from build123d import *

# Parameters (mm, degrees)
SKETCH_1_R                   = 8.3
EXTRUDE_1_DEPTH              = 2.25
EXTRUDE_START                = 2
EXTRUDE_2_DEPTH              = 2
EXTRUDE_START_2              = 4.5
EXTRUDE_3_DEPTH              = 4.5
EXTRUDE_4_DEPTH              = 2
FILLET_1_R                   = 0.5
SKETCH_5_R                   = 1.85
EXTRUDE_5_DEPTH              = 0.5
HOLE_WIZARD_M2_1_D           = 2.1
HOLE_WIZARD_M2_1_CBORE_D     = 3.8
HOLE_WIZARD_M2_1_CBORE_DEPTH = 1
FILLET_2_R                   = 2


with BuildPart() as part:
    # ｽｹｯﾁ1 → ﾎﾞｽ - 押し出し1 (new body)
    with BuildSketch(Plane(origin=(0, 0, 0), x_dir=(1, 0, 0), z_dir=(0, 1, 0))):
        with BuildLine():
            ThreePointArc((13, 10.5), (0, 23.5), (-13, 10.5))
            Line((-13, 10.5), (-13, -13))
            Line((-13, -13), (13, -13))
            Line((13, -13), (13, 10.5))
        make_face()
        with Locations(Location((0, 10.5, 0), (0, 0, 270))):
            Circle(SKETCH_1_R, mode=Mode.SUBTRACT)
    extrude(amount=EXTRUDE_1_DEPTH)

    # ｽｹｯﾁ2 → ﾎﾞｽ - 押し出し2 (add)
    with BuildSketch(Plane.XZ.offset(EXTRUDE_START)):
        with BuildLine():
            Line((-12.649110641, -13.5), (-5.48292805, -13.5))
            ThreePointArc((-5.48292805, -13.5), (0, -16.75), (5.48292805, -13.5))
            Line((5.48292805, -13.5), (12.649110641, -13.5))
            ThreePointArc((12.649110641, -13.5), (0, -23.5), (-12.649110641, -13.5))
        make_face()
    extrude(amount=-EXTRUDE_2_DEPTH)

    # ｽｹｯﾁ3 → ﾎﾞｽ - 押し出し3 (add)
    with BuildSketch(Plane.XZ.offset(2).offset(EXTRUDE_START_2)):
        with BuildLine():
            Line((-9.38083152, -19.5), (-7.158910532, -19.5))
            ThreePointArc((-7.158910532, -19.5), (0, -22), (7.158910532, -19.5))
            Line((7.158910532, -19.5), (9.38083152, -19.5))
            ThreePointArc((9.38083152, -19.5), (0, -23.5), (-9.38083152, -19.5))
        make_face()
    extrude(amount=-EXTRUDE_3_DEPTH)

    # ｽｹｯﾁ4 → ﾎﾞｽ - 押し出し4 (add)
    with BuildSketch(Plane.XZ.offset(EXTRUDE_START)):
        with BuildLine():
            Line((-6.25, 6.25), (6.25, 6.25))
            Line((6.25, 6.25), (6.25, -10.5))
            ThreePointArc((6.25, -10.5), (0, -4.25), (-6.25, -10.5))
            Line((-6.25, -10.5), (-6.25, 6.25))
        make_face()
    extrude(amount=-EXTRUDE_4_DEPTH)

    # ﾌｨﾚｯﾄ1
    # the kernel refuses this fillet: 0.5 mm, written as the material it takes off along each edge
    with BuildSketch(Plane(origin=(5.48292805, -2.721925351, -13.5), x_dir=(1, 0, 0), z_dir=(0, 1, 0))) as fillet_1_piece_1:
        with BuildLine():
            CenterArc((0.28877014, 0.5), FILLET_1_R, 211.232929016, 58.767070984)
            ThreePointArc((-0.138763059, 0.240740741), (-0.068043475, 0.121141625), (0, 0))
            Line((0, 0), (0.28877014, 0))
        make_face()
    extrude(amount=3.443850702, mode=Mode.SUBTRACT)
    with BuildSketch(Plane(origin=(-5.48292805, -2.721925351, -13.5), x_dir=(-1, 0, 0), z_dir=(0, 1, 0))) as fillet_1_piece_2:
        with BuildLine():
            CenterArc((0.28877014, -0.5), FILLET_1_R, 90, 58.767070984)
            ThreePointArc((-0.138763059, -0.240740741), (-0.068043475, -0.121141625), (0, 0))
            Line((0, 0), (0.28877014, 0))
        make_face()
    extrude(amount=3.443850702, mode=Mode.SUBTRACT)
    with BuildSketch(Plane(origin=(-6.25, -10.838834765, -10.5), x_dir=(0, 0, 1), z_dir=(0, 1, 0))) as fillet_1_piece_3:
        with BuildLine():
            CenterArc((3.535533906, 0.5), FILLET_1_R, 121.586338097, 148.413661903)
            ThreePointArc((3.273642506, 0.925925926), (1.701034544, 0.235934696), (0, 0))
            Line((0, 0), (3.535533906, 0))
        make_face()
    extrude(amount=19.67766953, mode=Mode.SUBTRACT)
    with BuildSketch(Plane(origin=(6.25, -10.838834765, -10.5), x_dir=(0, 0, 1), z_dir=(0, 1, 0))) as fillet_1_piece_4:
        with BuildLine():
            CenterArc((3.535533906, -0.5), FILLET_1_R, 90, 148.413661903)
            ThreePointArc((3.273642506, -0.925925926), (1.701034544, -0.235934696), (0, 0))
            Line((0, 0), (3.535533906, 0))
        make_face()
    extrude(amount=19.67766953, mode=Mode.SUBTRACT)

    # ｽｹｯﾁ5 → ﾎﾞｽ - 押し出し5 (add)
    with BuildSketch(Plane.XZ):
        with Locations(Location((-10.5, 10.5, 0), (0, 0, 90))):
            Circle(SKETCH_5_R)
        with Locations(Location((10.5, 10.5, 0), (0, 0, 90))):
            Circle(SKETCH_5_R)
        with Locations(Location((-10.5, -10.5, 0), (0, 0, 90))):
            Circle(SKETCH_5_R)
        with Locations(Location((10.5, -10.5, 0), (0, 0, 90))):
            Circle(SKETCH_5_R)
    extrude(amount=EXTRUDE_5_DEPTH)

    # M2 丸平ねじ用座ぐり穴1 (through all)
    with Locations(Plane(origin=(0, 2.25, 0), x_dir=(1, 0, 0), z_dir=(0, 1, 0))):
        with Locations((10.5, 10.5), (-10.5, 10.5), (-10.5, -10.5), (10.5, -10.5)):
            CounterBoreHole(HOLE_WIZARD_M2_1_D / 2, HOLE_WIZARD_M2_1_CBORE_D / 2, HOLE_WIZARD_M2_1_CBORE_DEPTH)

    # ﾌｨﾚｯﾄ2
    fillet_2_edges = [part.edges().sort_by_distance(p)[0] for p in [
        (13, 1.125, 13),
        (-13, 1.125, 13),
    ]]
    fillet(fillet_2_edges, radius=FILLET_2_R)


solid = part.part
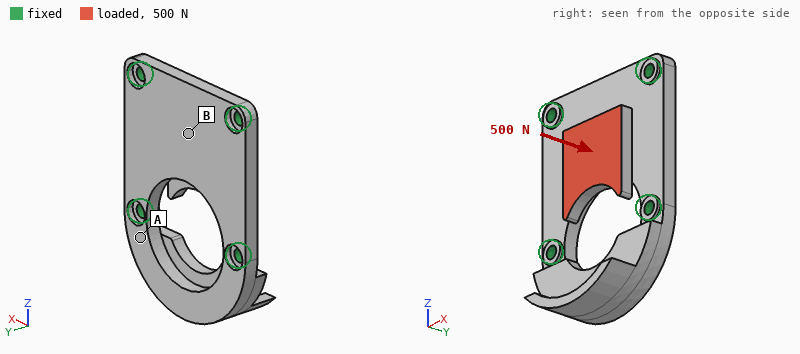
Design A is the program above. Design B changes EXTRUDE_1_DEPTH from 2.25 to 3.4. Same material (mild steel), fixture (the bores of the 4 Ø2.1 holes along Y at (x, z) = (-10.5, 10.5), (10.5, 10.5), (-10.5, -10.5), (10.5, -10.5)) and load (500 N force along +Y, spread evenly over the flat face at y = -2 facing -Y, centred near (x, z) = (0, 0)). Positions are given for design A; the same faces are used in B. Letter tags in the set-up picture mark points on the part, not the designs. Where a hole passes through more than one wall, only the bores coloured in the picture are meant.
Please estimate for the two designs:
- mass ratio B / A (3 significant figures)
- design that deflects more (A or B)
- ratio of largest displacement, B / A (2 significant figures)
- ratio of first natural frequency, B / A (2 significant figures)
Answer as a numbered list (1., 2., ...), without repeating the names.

1. 1.32
2. A
3. 0.48
4. 1.3
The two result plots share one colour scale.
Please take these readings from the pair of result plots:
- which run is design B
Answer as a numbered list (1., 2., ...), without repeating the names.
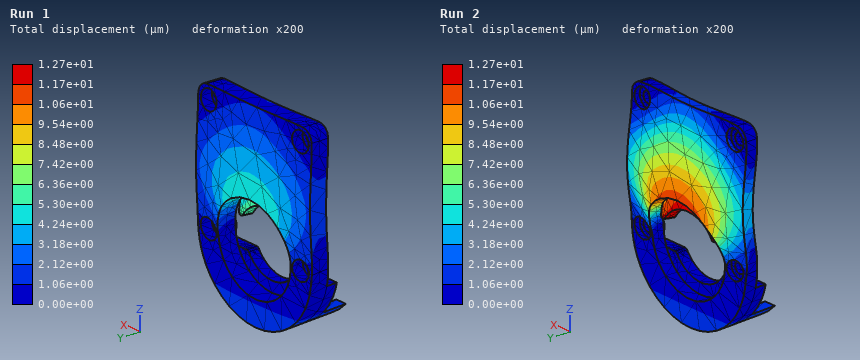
1. Run 1
